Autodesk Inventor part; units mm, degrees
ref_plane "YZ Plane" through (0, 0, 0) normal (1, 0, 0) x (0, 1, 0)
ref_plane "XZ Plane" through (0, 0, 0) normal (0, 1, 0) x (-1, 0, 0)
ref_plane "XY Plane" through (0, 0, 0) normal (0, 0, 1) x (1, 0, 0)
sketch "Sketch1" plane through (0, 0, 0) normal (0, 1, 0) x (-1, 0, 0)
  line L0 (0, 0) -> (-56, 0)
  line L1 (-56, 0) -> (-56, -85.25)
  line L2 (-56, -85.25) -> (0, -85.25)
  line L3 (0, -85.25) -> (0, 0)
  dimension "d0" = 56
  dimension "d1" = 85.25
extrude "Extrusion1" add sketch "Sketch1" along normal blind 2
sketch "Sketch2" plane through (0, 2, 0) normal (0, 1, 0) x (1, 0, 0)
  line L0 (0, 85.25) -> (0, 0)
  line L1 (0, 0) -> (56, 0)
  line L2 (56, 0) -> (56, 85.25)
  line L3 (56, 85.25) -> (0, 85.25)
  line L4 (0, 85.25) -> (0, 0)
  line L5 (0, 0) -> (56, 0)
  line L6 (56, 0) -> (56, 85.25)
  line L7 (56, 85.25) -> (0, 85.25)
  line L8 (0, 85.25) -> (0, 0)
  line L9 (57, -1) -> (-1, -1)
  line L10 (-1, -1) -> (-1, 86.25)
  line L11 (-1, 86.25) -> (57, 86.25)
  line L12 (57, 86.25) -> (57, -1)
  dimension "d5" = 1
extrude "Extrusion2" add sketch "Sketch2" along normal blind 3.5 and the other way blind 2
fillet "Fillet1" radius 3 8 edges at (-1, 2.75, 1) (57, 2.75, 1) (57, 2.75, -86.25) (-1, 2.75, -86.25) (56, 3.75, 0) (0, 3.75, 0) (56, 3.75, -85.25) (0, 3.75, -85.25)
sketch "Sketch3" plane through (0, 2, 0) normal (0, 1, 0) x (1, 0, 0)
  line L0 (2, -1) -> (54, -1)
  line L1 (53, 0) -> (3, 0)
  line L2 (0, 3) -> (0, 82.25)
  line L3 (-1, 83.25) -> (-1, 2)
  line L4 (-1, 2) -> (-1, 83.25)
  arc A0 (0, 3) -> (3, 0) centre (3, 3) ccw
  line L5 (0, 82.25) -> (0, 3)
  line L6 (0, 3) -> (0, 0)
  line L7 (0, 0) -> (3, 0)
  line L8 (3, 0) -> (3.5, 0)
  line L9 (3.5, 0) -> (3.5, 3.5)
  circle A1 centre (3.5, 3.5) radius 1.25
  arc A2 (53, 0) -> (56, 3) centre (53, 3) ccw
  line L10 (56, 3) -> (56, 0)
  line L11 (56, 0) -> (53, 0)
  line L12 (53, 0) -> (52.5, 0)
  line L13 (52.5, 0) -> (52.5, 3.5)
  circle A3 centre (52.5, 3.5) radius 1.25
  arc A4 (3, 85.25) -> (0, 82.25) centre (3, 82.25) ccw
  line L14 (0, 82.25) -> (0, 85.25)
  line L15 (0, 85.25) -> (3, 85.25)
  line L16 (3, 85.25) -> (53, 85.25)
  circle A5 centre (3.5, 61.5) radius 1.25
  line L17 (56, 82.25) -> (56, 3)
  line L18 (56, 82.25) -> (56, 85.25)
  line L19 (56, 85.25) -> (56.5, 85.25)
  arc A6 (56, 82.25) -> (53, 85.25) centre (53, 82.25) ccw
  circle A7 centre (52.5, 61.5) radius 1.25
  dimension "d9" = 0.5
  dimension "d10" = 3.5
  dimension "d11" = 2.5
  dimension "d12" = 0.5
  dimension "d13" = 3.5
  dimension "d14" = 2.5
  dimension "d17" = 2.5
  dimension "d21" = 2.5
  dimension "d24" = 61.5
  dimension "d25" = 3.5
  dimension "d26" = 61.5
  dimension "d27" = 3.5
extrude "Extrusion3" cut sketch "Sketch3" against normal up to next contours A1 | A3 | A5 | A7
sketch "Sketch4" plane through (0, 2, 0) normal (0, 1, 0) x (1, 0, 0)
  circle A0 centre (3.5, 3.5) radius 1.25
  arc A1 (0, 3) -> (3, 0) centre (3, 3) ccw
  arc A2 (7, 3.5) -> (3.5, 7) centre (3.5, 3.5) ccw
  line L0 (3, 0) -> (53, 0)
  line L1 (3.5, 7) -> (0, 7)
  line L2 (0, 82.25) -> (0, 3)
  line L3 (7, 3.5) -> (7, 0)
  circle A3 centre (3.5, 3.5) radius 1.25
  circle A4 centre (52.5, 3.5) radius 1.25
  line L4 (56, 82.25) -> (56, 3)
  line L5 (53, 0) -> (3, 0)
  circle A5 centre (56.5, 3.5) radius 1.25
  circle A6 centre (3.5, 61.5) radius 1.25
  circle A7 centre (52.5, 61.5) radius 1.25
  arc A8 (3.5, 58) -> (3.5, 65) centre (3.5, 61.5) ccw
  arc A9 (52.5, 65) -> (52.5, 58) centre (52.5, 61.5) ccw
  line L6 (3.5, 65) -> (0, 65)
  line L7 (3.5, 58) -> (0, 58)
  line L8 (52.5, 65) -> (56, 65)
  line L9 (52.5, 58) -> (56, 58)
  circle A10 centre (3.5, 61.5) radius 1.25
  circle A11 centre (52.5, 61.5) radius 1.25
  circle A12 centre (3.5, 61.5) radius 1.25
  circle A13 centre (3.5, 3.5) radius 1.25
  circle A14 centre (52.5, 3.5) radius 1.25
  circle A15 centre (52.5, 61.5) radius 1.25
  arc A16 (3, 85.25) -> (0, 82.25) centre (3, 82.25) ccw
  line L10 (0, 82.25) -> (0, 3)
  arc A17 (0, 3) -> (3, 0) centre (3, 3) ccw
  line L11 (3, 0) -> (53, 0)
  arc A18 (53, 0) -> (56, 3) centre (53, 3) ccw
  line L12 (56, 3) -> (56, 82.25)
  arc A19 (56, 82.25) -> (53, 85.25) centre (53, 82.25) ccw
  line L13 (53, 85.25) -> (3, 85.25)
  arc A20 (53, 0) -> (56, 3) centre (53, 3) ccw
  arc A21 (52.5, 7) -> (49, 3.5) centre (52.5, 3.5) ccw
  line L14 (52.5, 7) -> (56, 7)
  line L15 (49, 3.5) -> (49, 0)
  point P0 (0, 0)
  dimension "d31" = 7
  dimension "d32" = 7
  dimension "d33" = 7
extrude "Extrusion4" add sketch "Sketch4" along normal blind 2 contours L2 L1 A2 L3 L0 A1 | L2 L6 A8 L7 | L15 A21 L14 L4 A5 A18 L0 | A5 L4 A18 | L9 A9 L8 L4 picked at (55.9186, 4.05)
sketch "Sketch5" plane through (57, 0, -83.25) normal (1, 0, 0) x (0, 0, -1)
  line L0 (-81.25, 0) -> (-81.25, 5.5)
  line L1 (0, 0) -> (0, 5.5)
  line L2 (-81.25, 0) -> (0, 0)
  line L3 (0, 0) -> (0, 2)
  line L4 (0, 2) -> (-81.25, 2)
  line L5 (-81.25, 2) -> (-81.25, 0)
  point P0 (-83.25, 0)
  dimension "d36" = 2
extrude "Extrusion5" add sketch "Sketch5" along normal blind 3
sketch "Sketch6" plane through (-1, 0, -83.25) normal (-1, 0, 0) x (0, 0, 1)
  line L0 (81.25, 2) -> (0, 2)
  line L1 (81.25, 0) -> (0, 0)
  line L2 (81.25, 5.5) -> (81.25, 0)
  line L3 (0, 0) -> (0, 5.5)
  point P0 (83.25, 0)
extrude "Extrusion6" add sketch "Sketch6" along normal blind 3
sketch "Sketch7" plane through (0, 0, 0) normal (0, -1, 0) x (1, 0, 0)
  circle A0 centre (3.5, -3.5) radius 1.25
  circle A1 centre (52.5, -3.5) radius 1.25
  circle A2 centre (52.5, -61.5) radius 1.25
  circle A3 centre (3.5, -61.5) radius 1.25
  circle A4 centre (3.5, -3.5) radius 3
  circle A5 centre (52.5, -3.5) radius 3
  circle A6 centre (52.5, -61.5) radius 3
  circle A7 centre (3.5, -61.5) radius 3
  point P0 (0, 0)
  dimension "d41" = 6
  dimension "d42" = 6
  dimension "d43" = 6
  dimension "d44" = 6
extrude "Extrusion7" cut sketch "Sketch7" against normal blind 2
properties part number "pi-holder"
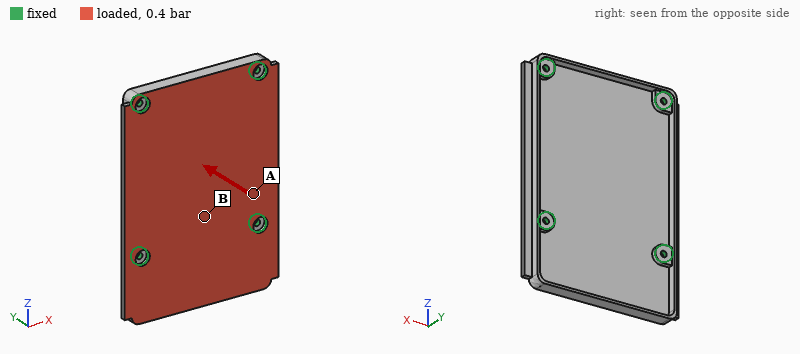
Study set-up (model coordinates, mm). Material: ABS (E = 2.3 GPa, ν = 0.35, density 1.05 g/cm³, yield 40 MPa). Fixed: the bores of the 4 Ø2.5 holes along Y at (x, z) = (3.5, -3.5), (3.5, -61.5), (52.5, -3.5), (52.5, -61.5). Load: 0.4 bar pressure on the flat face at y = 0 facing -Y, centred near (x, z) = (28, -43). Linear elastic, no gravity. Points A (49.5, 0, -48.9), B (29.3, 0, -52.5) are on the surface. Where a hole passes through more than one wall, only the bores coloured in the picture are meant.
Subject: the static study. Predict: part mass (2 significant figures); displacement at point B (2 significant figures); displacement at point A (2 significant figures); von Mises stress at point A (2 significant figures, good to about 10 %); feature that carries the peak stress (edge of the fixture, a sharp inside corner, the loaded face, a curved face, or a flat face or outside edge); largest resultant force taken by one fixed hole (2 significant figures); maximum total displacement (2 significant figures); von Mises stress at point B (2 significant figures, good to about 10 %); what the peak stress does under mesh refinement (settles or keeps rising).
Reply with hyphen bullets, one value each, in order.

- 13 g
- 0.74 mm
- 0.30 mm
- 3.2 MPa
- edge of the fixture
- 110 N
- 1.0 mm
- 8.2 MPa
- keeps rising
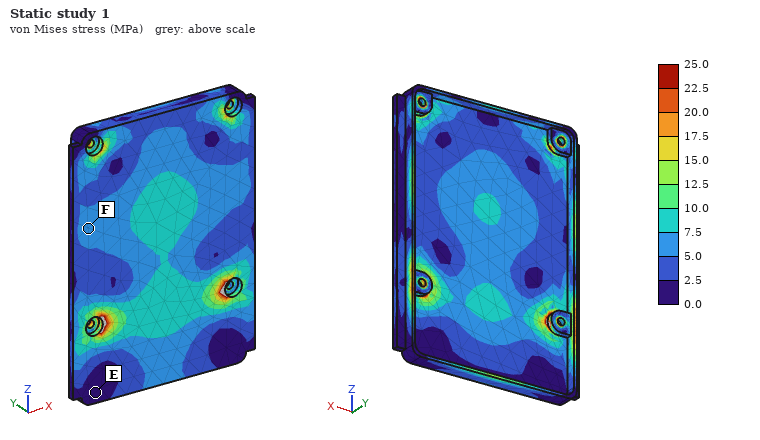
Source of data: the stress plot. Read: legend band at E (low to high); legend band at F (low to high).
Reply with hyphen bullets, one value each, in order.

- 0.0 to 2.5 MPa
- 5.0 to 7.5 MPa
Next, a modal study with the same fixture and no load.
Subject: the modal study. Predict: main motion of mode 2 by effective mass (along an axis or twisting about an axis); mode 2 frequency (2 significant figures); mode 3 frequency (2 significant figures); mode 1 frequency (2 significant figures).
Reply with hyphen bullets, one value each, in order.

- along Y
- 830 Hz
- 1200 Hz
- 690 Hz
